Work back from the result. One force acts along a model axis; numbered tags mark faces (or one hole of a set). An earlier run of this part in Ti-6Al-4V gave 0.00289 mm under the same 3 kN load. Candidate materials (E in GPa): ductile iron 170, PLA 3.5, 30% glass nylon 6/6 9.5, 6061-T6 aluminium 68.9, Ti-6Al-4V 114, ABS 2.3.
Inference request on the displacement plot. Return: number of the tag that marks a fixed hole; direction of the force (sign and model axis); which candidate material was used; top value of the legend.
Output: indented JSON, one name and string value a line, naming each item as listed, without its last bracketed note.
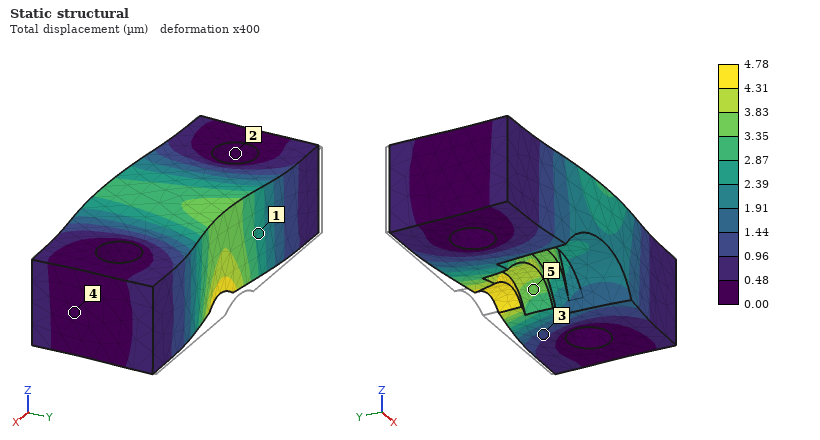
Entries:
{
  "number of the tag that marks a fixed hole": "2",
  "direction of the force": "-Y",
  "which candidate material was used": "6061-T6 aluminium",
  "top value of the legend": "4.78 µm"
}
